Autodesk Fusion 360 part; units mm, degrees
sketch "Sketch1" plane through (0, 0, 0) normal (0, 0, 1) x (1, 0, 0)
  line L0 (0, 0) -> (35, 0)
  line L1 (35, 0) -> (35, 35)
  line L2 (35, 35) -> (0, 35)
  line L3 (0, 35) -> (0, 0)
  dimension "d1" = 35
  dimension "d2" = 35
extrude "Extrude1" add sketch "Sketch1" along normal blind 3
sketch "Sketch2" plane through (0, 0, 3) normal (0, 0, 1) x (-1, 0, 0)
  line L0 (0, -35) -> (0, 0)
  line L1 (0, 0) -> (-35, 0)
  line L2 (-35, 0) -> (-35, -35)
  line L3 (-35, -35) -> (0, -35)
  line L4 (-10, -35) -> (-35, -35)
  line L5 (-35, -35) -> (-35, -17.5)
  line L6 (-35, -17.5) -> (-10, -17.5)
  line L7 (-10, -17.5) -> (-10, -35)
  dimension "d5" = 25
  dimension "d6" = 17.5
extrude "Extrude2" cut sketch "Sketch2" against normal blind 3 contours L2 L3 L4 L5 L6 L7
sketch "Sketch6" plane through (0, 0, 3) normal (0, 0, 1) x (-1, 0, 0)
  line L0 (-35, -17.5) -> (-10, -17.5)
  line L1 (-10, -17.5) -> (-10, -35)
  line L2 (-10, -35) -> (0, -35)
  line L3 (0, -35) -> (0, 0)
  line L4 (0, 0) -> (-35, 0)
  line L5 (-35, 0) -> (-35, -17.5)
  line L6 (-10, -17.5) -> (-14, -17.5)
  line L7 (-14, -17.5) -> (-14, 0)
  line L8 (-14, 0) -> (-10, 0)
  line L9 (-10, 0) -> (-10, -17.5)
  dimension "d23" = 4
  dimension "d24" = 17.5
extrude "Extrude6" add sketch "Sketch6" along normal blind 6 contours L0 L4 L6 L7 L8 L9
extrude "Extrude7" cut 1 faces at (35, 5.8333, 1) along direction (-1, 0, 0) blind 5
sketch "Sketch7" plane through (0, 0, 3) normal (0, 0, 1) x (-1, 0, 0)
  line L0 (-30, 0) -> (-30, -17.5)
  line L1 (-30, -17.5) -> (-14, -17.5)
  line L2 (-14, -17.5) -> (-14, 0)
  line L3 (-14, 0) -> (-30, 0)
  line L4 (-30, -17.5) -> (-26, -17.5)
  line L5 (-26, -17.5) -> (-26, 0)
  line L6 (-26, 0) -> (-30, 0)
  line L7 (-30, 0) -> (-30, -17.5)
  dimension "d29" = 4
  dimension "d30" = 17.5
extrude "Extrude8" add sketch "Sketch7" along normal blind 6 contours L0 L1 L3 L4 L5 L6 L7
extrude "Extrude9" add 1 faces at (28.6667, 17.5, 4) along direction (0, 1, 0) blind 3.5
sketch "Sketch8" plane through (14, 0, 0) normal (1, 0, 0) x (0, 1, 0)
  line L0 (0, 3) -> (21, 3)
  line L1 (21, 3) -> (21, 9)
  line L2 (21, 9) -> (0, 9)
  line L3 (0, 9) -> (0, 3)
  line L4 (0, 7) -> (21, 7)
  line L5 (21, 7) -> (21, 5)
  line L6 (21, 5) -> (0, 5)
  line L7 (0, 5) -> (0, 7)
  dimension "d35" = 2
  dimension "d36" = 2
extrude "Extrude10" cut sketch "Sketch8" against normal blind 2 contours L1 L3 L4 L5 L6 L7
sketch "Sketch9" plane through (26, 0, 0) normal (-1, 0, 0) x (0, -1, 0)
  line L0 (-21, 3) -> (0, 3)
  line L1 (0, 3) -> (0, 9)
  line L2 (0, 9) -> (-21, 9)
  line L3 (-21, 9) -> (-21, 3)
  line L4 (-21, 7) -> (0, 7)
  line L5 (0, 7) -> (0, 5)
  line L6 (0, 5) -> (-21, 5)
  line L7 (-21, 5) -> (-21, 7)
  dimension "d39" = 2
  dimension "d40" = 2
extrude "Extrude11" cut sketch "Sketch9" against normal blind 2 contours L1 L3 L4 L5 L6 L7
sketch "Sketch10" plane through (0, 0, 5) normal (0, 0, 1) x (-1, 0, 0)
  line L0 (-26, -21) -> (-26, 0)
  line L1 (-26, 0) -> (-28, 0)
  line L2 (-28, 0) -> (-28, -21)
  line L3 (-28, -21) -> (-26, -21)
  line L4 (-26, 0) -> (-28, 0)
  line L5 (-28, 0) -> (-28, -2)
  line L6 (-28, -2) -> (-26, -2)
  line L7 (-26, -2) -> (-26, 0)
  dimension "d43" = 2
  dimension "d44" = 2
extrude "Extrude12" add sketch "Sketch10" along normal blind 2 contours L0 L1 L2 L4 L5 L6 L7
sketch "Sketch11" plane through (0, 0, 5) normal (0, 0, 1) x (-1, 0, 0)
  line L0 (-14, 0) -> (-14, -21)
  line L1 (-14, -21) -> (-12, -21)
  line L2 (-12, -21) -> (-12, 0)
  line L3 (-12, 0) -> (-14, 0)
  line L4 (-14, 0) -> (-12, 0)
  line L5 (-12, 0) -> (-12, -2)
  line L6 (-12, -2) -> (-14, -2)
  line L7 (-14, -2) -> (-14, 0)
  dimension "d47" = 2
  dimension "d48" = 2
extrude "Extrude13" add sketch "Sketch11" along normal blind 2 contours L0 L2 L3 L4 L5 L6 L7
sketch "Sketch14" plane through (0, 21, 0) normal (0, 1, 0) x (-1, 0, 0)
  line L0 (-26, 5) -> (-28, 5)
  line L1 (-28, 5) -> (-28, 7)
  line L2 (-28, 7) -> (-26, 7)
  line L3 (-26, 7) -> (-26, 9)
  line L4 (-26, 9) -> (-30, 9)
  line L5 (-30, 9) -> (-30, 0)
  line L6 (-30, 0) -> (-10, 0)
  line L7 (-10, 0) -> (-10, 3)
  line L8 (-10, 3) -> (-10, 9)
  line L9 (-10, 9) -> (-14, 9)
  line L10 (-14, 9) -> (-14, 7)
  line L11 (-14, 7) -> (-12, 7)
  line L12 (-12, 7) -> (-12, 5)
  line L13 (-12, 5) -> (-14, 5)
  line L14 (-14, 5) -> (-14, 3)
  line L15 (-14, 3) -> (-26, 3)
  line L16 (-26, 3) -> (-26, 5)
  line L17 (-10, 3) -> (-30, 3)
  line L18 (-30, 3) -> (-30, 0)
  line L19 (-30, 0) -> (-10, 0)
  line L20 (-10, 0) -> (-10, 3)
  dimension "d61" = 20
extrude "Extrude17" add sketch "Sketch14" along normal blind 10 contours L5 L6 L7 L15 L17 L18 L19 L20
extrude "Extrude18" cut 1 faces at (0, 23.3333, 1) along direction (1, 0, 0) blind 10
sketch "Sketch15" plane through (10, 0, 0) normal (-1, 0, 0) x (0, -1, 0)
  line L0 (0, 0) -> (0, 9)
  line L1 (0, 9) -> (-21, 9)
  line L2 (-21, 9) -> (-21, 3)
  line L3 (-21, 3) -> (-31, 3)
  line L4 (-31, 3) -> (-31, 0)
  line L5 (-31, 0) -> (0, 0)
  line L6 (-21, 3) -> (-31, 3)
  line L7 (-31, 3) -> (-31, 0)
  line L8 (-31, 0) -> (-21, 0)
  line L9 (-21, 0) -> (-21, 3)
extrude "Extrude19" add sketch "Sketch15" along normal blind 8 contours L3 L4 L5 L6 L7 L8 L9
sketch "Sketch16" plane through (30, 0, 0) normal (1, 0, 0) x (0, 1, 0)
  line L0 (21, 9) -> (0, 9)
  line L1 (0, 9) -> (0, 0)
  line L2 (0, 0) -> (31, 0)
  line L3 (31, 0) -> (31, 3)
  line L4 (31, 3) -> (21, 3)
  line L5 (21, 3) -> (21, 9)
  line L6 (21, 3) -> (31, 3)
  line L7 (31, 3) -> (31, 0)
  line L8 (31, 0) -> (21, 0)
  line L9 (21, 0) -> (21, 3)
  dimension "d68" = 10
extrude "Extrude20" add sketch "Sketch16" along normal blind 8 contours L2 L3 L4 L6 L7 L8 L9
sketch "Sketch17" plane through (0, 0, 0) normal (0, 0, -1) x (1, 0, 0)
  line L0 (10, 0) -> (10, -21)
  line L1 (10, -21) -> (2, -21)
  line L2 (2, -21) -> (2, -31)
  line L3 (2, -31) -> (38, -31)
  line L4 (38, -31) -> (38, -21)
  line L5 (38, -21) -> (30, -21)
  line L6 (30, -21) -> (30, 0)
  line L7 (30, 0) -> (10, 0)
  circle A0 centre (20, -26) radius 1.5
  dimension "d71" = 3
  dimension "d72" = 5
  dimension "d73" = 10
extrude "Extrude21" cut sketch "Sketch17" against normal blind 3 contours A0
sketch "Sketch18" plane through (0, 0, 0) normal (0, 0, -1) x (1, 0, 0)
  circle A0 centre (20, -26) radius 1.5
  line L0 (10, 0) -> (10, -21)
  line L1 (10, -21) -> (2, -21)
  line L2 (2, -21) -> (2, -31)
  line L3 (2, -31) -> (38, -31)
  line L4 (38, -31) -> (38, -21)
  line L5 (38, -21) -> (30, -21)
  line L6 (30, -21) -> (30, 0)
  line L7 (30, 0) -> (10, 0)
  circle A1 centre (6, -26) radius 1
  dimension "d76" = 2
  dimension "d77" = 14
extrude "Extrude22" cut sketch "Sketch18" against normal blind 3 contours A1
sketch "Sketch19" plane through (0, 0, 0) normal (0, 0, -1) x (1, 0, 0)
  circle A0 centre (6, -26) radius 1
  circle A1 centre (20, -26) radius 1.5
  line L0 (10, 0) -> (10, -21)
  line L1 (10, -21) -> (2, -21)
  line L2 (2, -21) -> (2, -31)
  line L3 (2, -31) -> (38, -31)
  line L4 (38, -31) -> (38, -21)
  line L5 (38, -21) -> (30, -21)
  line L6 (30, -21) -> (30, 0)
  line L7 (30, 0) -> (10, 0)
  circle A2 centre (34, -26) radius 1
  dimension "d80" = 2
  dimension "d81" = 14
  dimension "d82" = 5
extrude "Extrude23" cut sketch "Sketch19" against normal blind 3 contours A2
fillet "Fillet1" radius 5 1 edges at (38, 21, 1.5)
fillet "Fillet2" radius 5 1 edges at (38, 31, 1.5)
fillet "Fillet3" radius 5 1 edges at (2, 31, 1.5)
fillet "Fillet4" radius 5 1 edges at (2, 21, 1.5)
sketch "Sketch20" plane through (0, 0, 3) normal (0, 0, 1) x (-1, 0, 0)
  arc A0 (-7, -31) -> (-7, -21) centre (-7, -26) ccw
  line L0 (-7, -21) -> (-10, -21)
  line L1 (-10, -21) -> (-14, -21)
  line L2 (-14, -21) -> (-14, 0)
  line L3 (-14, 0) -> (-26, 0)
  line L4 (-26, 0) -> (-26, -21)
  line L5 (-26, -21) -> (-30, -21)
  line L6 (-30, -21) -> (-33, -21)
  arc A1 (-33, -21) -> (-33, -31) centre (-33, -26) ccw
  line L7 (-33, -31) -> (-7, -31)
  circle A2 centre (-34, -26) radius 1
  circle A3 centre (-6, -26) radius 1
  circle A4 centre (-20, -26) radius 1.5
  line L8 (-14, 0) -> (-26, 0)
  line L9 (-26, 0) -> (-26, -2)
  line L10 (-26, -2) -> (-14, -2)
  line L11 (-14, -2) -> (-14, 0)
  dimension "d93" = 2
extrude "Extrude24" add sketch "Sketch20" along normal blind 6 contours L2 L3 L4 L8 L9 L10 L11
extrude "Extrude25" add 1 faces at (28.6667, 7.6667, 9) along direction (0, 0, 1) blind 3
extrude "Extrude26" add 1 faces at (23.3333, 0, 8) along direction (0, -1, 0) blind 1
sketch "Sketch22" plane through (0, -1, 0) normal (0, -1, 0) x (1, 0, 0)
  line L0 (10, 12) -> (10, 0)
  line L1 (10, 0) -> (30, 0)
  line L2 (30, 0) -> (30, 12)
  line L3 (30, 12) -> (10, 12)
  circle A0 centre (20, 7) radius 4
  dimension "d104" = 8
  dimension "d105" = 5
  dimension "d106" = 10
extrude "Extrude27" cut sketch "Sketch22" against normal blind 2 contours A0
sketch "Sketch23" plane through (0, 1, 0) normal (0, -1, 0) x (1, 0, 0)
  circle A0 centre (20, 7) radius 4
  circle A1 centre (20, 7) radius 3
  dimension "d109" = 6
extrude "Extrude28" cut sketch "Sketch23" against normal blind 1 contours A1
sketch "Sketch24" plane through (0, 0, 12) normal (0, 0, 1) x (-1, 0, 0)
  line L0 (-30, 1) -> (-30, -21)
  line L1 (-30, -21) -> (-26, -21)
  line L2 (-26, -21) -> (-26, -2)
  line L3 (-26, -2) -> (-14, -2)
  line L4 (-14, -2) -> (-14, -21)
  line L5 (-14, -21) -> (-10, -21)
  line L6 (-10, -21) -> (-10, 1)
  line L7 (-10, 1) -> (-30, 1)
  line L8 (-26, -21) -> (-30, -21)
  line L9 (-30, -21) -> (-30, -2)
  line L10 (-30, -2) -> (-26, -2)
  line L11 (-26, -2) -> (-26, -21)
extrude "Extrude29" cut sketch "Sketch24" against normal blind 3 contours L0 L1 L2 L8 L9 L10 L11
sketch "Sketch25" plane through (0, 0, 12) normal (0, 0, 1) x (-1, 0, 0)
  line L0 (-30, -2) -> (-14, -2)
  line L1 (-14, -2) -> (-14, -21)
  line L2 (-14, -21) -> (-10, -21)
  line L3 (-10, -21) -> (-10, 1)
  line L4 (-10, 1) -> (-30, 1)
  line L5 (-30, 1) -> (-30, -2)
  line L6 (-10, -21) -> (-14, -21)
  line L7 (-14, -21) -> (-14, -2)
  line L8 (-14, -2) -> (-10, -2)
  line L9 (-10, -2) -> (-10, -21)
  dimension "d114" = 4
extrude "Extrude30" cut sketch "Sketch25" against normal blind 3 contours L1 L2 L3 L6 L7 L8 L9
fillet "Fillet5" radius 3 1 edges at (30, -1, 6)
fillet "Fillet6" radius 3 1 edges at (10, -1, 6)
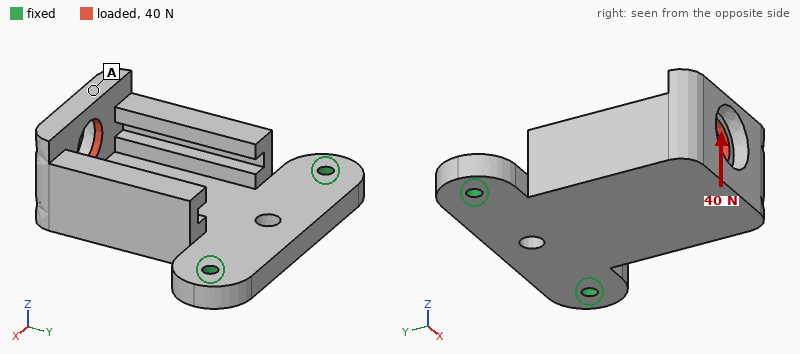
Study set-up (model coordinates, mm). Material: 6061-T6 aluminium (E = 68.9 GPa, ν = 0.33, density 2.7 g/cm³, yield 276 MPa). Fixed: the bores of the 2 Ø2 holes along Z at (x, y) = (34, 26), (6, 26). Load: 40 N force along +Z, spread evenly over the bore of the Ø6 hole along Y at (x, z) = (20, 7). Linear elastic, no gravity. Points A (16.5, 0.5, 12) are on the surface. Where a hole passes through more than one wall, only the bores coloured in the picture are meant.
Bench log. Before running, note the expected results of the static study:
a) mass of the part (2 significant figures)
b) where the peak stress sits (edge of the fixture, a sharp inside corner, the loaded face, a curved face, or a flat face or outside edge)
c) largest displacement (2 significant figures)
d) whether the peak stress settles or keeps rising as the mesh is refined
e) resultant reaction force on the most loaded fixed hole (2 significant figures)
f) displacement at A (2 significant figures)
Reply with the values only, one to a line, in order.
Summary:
9.2 g
edge of the fixture
85 µm
keeps rising
20 N
80 µm
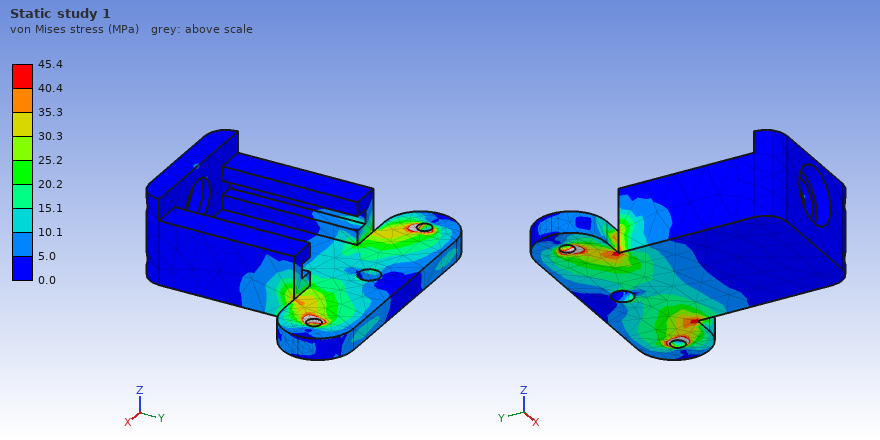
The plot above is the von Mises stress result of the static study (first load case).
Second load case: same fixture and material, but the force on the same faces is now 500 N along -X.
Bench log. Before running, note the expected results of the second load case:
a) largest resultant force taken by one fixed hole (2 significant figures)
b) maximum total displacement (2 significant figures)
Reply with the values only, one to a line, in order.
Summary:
530 N
98 µm
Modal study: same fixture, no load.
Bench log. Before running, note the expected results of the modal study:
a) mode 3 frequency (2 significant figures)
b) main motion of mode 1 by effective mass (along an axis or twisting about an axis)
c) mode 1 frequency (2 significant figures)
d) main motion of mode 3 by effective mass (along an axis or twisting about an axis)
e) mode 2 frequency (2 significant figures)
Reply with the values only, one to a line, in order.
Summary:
12 kHz
along Z
2000 Hz
along X
7200 Hz
